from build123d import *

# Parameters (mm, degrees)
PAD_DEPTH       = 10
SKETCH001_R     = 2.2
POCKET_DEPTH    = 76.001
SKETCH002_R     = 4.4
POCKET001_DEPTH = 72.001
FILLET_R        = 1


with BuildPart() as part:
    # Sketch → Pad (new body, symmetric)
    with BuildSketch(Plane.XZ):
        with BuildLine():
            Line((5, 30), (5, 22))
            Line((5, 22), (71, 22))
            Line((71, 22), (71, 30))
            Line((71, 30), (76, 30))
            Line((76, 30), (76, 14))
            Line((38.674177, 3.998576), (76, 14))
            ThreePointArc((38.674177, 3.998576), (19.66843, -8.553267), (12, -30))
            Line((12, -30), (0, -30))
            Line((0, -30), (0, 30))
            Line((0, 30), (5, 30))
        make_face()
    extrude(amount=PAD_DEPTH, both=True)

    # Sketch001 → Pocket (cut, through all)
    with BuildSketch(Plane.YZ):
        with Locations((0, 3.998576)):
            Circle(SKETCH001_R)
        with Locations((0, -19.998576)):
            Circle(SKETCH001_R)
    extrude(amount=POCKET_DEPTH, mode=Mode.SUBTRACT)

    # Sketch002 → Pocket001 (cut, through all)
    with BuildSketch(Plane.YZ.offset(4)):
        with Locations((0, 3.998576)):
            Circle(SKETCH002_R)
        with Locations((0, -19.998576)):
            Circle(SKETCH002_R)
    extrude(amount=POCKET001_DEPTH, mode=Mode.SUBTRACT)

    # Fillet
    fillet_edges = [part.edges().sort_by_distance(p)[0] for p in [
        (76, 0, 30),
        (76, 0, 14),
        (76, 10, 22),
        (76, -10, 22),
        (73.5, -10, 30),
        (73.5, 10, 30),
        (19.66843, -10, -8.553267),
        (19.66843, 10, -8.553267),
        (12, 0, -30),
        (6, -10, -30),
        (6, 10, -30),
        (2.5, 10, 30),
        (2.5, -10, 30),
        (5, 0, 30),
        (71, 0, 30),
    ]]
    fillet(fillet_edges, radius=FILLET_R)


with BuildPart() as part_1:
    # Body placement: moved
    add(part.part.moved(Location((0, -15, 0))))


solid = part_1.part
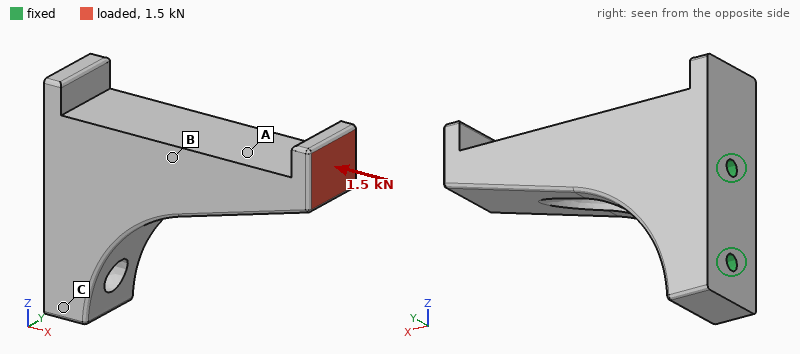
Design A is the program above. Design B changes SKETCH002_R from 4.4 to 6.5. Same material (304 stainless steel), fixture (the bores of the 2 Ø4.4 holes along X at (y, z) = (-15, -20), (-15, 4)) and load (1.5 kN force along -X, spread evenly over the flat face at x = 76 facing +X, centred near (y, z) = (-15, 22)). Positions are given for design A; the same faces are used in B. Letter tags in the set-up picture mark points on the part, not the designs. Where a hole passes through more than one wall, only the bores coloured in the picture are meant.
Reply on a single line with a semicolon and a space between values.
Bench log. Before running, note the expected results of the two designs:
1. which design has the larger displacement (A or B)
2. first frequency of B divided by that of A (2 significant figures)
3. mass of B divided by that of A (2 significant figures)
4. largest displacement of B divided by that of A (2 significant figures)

B; 0.95; 0.90; 1.2
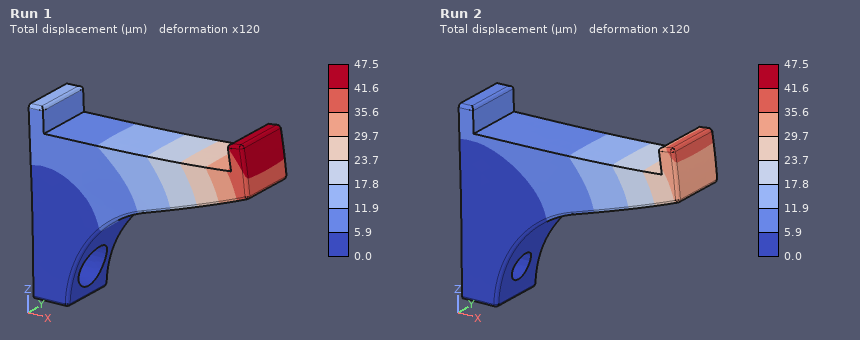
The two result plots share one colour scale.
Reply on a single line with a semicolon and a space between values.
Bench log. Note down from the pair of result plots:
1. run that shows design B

Run 1
